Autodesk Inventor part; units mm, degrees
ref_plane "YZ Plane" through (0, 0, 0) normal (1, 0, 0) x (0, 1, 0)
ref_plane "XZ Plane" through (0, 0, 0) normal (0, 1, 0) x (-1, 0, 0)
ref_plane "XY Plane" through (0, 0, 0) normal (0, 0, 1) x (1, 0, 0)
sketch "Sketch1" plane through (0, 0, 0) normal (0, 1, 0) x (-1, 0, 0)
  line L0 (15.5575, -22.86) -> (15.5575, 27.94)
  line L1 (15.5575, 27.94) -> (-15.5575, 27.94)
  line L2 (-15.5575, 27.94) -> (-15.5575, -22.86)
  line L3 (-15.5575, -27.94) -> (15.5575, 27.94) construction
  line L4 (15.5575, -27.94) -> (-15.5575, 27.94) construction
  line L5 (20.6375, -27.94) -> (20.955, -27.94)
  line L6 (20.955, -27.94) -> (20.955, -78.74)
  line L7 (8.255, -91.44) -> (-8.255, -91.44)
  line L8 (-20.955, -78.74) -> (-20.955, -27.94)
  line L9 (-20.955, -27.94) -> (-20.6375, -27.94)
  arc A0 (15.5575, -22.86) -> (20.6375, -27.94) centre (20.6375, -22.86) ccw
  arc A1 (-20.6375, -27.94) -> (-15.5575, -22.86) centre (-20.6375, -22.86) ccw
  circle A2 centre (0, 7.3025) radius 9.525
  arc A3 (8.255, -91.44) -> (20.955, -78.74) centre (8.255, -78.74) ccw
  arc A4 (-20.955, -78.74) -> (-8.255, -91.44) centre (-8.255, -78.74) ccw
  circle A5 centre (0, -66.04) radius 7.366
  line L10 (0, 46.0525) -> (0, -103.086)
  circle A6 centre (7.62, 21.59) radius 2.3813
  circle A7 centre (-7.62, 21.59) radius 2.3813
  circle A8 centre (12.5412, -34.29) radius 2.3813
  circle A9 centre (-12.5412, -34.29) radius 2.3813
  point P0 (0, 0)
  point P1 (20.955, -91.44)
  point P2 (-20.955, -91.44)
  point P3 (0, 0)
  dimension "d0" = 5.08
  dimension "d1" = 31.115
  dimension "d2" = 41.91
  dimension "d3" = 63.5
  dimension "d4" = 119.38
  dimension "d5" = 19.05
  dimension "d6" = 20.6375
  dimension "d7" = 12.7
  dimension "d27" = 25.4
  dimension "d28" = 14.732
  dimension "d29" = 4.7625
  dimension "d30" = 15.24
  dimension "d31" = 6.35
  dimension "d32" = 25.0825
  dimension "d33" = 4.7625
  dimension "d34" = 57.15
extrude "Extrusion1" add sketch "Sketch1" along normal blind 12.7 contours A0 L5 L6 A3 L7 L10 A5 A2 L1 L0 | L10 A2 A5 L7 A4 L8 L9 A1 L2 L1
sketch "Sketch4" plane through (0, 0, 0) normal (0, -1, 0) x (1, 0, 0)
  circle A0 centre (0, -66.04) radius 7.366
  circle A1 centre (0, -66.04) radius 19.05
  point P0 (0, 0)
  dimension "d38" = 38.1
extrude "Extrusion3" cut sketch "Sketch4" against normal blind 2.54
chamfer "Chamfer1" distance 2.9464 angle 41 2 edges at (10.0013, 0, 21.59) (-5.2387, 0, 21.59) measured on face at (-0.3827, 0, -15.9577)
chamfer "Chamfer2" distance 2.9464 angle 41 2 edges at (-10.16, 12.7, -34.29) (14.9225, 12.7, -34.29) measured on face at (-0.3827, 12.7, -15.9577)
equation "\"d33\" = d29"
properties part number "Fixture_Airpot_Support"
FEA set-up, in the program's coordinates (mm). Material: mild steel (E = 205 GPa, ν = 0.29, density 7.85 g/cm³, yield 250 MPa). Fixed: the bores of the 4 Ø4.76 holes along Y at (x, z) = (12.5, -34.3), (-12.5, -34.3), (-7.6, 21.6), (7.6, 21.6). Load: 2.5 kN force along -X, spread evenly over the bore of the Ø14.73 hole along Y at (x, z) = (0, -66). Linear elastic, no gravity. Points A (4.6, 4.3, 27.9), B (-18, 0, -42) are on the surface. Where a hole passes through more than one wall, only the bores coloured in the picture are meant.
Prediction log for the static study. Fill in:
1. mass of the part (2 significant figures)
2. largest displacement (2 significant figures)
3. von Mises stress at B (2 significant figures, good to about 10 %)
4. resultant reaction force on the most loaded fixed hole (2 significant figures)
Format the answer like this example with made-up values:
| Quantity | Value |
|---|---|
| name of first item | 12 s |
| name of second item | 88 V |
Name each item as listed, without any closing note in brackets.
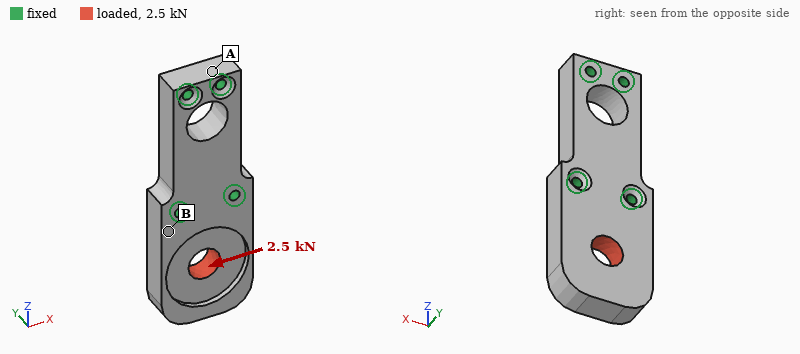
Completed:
| Quantity | Value |
|---|---|
| mass of the part | 360 g |
| largest displacement | 9.3 µm |
| von Mises stress at B | 12 MPa |
| resultant reaction force on the most loaded fixed hole | 3.0 kN |
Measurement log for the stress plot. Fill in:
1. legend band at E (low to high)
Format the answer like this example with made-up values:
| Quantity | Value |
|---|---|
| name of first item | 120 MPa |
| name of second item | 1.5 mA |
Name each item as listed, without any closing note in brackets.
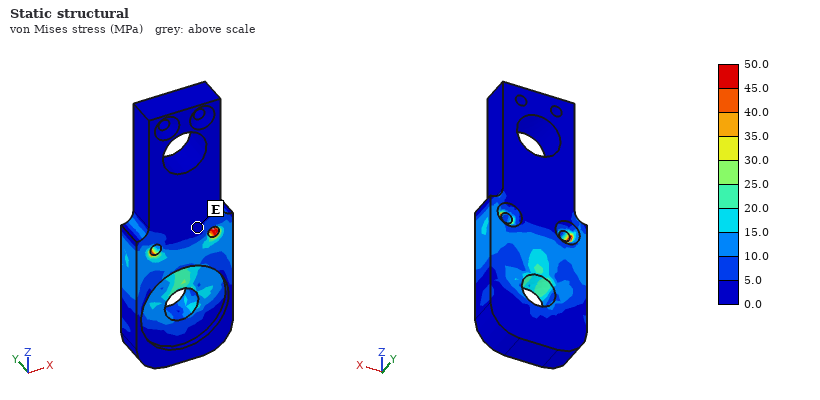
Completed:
| Quantity | Value |
|---|---|
| legend band at E | 0.0 to 5.0 MPa |
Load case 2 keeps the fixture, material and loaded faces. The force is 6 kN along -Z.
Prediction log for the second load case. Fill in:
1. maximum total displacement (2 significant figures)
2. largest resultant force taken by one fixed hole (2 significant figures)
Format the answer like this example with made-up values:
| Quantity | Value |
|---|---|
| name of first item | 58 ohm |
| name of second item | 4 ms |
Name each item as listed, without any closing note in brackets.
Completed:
| Quantity | Value |
|---|---|
| maximum total displacement | 8.4 µm |
| largest resultant force taken by one fixed hole | 2.9 kN |
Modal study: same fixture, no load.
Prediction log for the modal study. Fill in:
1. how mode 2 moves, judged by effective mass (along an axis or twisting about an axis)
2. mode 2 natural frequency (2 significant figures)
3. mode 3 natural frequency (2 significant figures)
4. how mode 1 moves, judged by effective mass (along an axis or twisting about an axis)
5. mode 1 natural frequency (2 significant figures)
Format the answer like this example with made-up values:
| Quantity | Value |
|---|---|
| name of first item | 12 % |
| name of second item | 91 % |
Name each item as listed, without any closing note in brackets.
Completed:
| Quantity | Value |
|---|---|
| how mode 2 moves, judged by effective mass | along X |
| mode 2 natural frequency | 6900 Hz |
| mode 3 natural frequency | 7800 Hz |
| how mode 1 moves, judged by effective mass | along Y |
| mode 1 natural frequency | 2800 Hz |
